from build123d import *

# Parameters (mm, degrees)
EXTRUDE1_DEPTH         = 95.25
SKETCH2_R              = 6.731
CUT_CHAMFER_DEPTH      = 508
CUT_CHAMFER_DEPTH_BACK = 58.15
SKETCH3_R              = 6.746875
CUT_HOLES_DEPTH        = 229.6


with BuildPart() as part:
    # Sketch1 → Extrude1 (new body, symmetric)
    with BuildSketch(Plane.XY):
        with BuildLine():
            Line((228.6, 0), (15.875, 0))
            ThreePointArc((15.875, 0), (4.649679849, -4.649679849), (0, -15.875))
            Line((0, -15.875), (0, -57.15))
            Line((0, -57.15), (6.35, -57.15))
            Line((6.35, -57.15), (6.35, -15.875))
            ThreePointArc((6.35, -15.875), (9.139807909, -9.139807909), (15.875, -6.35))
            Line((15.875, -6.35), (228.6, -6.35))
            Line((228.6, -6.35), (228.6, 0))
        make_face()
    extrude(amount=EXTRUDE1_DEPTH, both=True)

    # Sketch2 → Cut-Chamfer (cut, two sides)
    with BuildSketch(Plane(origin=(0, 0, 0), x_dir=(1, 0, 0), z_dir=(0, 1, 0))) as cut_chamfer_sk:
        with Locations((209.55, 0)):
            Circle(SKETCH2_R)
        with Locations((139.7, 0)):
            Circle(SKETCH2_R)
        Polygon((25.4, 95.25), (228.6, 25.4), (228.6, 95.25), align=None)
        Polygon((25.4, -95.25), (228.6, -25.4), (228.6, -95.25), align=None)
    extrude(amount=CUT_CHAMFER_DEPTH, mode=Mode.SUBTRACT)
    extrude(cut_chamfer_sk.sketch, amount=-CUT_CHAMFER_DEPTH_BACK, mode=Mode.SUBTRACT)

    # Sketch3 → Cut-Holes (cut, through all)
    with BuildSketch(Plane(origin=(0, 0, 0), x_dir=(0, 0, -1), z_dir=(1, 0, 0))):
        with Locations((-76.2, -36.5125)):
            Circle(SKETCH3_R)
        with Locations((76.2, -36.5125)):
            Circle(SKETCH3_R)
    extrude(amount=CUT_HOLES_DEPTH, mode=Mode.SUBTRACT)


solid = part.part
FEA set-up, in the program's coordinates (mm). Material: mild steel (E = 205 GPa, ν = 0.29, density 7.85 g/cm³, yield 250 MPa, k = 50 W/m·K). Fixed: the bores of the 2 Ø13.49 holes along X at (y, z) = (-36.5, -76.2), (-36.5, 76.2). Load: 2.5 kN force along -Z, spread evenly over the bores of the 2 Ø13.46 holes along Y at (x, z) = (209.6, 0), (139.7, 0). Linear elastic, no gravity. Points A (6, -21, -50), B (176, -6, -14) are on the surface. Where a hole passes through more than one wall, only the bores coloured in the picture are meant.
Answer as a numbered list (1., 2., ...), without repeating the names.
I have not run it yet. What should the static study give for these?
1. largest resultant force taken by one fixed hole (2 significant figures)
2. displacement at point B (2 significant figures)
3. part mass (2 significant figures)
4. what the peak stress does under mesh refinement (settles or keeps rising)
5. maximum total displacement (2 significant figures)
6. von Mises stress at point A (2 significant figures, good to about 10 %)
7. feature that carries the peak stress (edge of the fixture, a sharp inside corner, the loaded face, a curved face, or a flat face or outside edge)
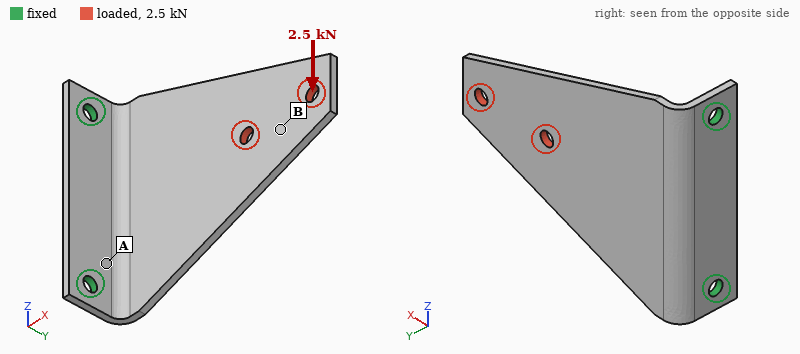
1. 3.1 kN
2. 0.20 mm
3. 1.9 kg
4. keeps rising
5. 0.27 mm
6. 52 MPa
7. edge of the fixture
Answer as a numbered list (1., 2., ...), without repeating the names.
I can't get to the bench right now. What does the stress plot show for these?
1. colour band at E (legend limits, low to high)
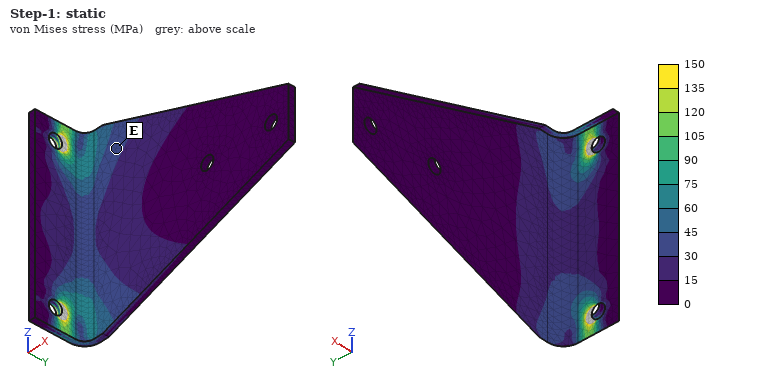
1. 30 to 45 MPa
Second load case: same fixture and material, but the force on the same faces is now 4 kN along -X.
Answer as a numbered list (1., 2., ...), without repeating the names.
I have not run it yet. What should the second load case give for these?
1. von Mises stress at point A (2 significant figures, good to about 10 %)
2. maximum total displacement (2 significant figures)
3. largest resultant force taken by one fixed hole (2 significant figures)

1. 46 MPa
2. 0.71 mm
3. 2.0 kN
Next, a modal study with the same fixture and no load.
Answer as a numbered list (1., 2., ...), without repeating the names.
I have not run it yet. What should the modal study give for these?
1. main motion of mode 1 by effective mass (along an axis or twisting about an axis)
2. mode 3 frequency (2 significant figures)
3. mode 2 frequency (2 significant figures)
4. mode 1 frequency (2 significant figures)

1. along Y
2. 590 Hz
3. 550 Hz
4. 120 Hz
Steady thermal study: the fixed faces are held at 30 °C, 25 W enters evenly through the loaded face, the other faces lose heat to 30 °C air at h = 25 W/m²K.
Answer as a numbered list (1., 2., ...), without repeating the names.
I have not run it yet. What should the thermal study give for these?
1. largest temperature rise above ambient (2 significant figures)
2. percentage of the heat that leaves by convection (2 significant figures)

1. 47 K
2. 90 %
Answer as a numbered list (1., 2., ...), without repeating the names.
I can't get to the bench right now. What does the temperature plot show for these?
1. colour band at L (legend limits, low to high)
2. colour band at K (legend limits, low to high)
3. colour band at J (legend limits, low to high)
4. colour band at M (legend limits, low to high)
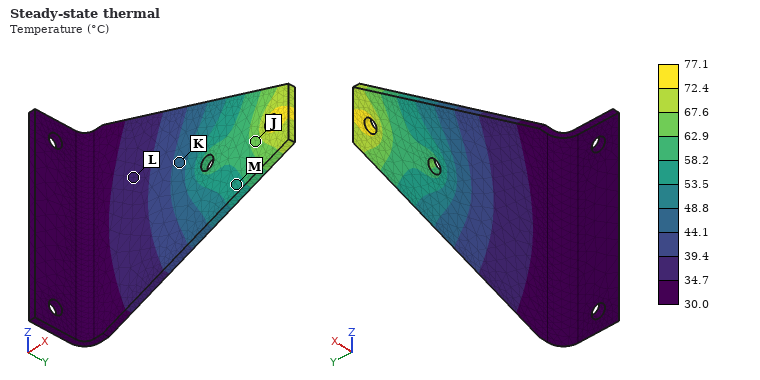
1. 34.7 to 39.4 °C
2. 44.1 to 48.8 °C
3. 62.9 to 67.6 °C
4. 53.5 to 58.2 °C
